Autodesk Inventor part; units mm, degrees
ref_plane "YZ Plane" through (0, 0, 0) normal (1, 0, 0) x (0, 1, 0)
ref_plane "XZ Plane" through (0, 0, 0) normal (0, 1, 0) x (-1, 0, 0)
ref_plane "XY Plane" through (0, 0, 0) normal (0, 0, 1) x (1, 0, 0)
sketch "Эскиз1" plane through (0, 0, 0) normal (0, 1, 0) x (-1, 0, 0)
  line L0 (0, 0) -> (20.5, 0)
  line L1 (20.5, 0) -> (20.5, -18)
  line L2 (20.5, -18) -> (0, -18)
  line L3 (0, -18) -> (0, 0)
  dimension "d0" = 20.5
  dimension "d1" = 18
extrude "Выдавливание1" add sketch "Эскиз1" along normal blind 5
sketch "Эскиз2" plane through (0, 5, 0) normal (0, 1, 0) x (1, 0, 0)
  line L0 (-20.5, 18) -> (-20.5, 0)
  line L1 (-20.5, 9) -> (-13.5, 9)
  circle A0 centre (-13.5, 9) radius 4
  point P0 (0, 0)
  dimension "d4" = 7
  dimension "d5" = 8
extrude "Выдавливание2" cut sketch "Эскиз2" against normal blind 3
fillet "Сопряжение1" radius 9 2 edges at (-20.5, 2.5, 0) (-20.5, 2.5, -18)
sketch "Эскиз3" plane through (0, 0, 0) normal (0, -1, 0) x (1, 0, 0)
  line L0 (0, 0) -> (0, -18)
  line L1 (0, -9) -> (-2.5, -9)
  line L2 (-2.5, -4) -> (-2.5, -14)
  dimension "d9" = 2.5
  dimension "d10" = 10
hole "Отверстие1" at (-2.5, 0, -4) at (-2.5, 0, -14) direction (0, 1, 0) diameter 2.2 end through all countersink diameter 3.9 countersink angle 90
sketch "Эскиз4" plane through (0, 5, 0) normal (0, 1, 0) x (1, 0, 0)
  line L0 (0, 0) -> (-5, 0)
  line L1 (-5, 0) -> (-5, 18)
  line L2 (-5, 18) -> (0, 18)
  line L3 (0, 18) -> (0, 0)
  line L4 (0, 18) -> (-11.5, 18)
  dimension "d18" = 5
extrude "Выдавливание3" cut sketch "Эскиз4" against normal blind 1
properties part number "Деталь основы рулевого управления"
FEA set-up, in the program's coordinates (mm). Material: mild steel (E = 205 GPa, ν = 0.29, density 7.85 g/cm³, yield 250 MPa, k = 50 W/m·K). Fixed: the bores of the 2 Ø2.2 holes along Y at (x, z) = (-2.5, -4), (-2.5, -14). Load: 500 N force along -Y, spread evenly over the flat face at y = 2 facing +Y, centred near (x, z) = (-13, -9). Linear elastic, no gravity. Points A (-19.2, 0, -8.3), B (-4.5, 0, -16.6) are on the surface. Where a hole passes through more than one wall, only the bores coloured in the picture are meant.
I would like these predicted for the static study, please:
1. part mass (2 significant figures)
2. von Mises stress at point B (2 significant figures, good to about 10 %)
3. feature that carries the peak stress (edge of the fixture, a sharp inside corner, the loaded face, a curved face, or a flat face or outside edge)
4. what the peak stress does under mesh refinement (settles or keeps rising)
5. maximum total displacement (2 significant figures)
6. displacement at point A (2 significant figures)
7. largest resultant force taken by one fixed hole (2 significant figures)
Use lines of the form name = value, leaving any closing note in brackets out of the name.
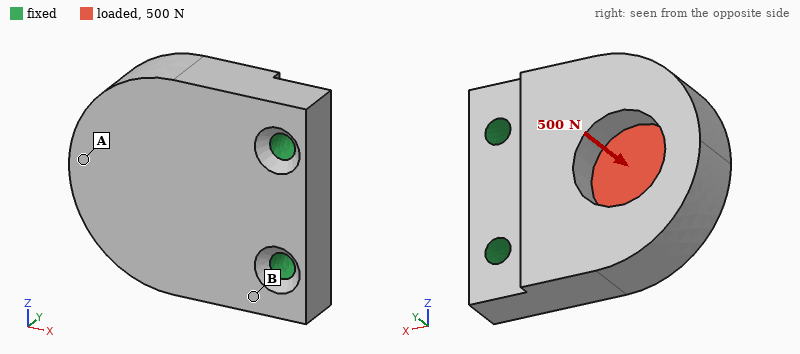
part mass = 11 g
von Mises stress at point B = 78 MPa
feature that carries the peak stress = edge of the fixture
what the peak stress does under mesh refinement = keeps rising
maximum total displacement = 27 µm
displacement at point A = 25 µm
largest resultant force taken by one fixed hole = 250 N
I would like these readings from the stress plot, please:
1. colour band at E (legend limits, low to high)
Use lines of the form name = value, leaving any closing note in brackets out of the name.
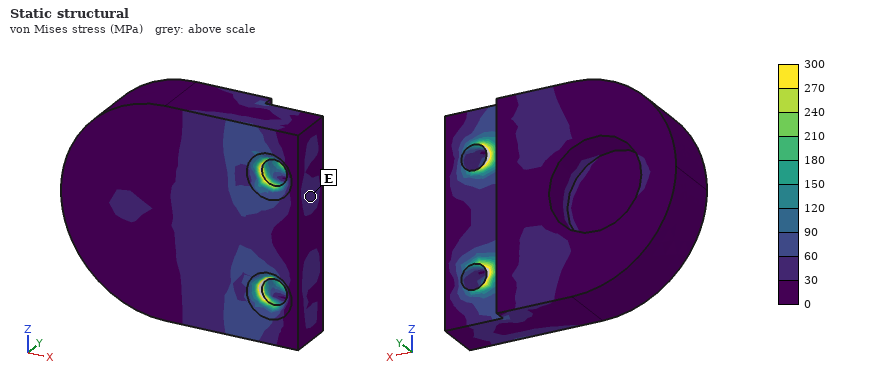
colour band at E = 30 to 60 MPa
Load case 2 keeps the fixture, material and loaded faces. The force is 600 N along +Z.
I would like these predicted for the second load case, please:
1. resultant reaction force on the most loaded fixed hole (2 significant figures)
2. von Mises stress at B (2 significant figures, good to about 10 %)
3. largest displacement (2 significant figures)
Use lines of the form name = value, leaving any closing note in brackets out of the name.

resultant reaction force on the most loaded fixed hole = 630 N
von Mises stress at B = 12 MPa
largest displacement = 3.7 µm
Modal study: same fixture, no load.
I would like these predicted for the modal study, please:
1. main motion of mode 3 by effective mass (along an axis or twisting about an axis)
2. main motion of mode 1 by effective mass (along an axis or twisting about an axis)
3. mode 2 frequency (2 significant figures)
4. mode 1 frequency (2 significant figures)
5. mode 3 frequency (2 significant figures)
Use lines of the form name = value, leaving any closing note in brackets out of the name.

main motion of mode 3 by effective mass = along Z
main motion of mode 1 by effective mass = along Y
mode 2 frequency = 26 kHz
mode 1 frequency = 11 kHz
mode 3 frequency = 29 kHz
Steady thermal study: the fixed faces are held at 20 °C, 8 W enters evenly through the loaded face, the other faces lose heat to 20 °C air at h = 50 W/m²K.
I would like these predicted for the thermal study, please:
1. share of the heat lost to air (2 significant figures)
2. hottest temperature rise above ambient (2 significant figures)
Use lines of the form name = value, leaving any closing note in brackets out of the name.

share of the heat lost to air = 8.4 %
hottest temperature rise above ambient = 31 K
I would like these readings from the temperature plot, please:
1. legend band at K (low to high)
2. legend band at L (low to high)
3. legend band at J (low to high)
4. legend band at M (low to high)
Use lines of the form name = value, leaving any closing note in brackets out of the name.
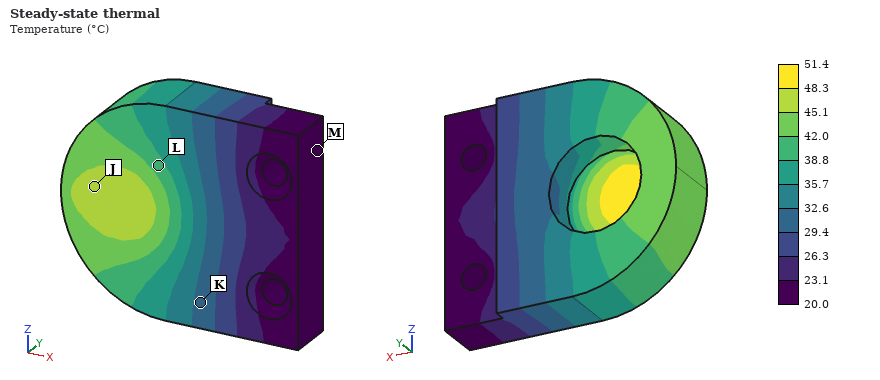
legend band at K = 29.4 to 32.6 °C
legend band at L = 38.8 to 42.0 °C
legend band at J = 45.1 to 48.3 °C
legend band at M = 20.0 to 23.1 °C
